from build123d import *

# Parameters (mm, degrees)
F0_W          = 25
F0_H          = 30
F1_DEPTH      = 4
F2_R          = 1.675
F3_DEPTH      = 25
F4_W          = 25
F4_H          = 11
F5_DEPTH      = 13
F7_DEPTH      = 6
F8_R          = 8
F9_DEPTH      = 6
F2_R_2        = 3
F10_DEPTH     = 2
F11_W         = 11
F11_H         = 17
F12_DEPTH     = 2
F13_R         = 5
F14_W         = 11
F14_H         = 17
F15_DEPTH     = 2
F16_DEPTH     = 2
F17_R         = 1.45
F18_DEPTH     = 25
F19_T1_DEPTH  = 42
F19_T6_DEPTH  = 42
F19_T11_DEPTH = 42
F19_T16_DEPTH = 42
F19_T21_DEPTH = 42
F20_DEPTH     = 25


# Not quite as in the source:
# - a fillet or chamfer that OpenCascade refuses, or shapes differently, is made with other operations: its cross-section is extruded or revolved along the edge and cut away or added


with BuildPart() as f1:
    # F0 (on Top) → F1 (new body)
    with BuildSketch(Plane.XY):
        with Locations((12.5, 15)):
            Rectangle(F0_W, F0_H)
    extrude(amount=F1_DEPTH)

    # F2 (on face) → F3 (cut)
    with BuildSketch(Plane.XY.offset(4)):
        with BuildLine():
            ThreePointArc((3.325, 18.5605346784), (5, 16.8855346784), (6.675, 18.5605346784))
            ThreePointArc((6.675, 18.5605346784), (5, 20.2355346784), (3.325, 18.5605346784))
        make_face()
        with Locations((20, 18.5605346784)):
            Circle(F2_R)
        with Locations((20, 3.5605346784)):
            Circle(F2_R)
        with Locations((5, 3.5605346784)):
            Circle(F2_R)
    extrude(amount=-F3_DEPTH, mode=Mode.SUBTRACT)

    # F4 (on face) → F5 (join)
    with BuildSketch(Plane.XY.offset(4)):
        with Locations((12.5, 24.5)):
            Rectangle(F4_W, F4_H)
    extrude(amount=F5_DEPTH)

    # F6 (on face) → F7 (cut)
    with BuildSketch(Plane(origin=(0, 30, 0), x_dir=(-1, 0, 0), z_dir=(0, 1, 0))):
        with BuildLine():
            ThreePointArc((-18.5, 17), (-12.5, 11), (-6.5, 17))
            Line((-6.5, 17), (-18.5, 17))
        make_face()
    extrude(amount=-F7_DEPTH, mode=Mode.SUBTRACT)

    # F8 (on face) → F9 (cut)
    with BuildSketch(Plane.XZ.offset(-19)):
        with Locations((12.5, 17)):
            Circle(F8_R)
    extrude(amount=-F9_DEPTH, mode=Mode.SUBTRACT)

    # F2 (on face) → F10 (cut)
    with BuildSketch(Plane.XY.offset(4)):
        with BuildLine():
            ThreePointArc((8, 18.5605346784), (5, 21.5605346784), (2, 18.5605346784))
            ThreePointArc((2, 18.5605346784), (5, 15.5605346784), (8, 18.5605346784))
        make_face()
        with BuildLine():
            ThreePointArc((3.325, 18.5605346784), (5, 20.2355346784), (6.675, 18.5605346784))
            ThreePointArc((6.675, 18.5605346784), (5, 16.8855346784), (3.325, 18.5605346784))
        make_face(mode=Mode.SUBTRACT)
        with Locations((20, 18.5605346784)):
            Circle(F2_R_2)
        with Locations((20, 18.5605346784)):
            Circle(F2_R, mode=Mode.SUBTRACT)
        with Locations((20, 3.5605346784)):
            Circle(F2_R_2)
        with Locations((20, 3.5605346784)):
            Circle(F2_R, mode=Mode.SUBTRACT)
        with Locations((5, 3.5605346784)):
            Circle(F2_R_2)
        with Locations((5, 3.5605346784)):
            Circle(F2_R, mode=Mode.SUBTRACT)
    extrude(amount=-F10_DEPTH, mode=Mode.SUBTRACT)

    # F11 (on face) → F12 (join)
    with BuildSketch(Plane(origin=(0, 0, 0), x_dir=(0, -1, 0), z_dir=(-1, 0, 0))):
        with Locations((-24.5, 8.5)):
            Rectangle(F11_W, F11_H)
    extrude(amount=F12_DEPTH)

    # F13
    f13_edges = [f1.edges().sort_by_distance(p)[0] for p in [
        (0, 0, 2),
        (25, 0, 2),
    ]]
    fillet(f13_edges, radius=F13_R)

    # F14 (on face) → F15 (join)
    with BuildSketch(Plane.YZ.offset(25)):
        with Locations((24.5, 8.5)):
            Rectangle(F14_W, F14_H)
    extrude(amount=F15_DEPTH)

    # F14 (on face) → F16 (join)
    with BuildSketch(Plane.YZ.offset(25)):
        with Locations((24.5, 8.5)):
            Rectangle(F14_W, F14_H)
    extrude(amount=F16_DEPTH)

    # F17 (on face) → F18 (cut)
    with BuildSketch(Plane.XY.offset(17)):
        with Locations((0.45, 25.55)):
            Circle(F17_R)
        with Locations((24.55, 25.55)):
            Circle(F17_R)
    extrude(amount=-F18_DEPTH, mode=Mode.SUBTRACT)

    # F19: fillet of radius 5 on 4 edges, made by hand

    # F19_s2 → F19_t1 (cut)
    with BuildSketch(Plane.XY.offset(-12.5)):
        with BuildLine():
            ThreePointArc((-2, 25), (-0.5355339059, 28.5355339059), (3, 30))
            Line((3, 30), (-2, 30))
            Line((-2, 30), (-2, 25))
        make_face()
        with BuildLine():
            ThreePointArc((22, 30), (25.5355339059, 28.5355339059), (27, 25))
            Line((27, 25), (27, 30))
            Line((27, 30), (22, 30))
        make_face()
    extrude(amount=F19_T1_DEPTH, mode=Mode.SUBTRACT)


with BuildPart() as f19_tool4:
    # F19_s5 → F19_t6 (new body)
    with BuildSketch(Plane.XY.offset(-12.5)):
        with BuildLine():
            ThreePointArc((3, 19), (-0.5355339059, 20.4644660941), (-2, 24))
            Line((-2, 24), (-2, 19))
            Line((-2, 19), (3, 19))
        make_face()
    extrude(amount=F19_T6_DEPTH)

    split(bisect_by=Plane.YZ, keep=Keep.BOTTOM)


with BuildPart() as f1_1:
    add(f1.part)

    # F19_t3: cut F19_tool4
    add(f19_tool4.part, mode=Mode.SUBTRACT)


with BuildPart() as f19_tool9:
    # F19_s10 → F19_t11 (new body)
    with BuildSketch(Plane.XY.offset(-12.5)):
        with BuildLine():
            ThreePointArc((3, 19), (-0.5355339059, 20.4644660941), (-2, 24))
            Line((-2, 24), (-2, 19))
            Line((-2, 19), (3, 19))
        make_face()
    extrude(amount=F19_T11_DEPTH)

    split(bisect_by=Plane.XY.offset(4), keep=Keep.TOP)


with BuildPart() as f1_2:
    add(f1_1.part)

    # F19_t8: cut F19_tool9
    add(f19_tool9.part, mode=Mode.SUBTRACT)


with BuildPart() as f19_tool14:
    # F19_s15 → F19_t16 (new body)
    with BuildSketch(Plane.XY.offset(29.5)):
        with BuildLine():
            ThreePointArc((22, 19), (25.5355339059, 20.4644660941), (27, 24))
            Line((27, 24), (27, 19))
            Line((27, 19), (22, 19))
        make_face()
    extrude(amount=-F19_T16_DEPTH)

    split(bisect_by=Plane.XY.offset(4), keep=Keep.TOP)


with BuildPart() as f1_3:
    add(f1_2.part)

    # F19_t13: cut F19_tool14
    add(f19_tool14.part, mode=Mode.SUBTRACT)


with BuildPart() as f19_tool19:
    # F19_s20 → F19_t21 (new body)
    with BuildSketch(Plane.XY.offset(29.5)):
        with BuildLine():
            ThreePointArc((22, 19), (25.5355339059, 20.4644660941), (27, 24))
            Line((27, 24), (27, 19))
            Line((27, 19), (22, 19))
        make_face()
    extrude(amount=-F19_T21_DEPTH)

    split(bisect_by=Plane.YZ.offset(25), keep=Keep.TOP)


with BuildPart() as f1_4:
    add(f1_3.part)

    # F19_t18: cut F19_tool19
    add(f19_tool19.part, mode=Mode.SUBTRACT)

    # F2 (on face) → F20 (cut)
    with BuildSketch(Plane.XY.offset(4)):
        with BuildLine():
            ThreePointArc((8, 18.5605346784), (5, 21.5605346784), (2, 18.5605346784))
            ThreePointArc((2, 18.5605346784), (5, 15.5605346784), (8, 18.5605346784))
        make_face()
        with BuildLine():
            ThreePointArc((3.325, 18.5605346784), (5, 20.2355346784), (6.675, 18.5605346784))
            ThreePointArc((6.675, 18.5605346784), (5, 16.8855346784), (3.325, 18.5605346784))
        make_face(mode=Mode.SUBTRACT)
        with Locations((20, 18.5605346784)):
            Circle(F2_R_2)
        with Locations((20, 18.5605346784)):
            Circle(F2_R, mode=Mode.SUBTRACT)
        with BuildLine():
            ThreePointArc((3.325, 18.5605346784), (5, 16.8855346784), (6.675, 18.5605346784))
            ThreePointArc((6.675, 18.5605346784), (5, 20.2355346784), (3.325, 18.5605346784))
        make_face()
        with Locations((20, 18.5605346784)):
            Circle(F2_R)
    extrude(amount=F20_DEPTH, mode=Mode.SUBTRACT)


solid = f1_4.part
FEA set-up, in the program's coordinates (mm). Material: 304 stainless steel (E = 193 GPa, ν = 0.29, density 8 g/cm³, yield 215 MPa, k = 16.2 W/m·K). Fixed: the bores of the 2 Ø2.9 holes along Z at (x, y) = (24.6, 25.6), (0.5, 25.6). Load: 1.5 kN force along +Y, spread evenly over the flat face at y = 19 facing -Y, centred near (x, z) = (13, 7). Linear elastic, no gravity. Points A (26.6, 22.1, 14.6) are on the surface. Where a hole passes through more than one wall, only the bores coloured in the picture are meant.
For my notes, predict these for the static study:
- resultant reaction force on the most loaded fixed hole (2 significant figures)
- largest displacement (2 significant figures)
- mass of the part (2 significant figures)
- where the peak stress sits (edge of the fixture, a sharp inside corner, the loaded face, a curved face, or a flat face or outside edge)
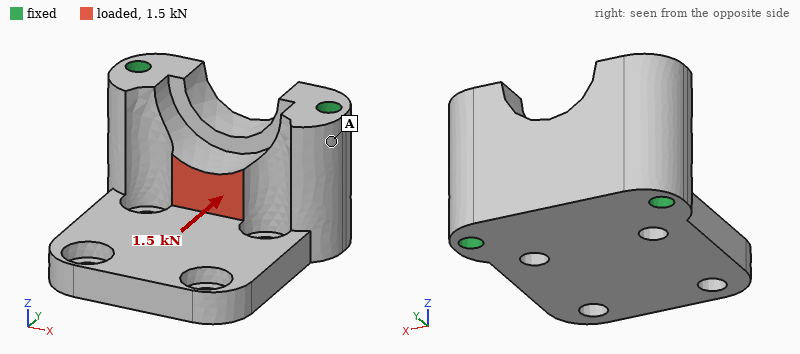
770 N
2.6 µm
42 g
a curved face
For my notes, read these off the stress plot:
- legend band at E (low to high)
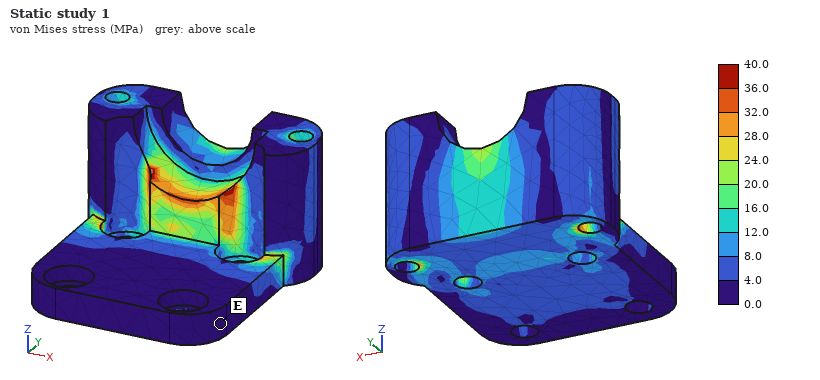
0.0 to 4.0 MPa
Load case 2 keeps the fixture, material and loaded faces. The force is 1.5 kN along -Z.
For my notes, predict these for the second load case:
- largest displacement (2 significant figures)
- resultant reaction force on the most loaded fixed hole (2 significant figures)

6.5 µm
770 N
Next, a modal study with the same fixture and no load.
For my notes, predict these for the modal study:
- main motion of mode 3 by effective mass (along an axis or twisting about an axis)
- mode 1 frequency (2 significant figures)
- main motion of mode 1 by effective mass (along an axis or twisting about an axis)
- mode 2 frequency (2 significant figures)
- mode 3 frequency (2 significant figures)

along X
6500 Hz
along Z
14 kHz
22 kHz
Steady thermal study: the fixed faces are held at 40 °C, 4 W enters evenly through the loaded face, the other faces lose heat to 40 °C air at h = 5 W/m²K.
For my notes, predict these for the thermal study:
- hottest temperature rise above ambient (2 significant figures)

26 K
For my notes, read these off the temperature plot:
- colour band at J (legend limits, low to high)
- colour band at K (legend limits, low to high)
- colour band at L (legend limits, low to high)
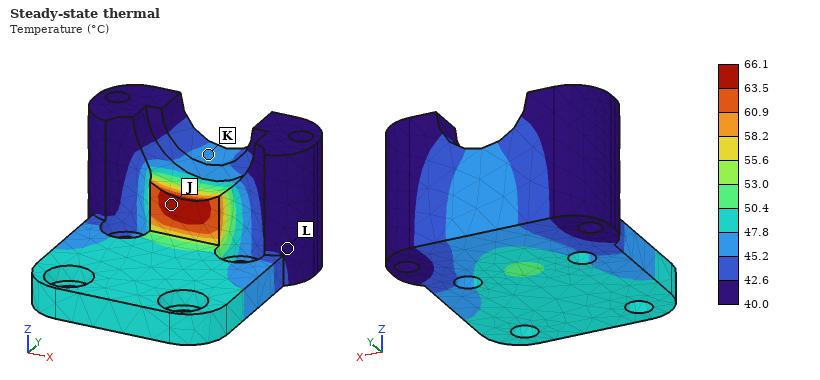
63.5 to 66.1 °C
45.2 to 47.8 °C
40.0 to 42.6 °C
